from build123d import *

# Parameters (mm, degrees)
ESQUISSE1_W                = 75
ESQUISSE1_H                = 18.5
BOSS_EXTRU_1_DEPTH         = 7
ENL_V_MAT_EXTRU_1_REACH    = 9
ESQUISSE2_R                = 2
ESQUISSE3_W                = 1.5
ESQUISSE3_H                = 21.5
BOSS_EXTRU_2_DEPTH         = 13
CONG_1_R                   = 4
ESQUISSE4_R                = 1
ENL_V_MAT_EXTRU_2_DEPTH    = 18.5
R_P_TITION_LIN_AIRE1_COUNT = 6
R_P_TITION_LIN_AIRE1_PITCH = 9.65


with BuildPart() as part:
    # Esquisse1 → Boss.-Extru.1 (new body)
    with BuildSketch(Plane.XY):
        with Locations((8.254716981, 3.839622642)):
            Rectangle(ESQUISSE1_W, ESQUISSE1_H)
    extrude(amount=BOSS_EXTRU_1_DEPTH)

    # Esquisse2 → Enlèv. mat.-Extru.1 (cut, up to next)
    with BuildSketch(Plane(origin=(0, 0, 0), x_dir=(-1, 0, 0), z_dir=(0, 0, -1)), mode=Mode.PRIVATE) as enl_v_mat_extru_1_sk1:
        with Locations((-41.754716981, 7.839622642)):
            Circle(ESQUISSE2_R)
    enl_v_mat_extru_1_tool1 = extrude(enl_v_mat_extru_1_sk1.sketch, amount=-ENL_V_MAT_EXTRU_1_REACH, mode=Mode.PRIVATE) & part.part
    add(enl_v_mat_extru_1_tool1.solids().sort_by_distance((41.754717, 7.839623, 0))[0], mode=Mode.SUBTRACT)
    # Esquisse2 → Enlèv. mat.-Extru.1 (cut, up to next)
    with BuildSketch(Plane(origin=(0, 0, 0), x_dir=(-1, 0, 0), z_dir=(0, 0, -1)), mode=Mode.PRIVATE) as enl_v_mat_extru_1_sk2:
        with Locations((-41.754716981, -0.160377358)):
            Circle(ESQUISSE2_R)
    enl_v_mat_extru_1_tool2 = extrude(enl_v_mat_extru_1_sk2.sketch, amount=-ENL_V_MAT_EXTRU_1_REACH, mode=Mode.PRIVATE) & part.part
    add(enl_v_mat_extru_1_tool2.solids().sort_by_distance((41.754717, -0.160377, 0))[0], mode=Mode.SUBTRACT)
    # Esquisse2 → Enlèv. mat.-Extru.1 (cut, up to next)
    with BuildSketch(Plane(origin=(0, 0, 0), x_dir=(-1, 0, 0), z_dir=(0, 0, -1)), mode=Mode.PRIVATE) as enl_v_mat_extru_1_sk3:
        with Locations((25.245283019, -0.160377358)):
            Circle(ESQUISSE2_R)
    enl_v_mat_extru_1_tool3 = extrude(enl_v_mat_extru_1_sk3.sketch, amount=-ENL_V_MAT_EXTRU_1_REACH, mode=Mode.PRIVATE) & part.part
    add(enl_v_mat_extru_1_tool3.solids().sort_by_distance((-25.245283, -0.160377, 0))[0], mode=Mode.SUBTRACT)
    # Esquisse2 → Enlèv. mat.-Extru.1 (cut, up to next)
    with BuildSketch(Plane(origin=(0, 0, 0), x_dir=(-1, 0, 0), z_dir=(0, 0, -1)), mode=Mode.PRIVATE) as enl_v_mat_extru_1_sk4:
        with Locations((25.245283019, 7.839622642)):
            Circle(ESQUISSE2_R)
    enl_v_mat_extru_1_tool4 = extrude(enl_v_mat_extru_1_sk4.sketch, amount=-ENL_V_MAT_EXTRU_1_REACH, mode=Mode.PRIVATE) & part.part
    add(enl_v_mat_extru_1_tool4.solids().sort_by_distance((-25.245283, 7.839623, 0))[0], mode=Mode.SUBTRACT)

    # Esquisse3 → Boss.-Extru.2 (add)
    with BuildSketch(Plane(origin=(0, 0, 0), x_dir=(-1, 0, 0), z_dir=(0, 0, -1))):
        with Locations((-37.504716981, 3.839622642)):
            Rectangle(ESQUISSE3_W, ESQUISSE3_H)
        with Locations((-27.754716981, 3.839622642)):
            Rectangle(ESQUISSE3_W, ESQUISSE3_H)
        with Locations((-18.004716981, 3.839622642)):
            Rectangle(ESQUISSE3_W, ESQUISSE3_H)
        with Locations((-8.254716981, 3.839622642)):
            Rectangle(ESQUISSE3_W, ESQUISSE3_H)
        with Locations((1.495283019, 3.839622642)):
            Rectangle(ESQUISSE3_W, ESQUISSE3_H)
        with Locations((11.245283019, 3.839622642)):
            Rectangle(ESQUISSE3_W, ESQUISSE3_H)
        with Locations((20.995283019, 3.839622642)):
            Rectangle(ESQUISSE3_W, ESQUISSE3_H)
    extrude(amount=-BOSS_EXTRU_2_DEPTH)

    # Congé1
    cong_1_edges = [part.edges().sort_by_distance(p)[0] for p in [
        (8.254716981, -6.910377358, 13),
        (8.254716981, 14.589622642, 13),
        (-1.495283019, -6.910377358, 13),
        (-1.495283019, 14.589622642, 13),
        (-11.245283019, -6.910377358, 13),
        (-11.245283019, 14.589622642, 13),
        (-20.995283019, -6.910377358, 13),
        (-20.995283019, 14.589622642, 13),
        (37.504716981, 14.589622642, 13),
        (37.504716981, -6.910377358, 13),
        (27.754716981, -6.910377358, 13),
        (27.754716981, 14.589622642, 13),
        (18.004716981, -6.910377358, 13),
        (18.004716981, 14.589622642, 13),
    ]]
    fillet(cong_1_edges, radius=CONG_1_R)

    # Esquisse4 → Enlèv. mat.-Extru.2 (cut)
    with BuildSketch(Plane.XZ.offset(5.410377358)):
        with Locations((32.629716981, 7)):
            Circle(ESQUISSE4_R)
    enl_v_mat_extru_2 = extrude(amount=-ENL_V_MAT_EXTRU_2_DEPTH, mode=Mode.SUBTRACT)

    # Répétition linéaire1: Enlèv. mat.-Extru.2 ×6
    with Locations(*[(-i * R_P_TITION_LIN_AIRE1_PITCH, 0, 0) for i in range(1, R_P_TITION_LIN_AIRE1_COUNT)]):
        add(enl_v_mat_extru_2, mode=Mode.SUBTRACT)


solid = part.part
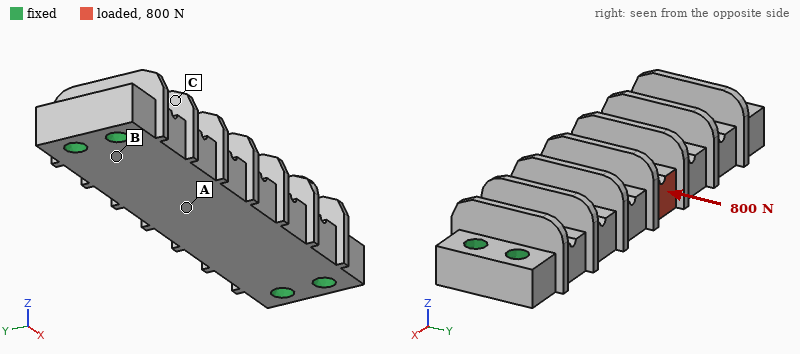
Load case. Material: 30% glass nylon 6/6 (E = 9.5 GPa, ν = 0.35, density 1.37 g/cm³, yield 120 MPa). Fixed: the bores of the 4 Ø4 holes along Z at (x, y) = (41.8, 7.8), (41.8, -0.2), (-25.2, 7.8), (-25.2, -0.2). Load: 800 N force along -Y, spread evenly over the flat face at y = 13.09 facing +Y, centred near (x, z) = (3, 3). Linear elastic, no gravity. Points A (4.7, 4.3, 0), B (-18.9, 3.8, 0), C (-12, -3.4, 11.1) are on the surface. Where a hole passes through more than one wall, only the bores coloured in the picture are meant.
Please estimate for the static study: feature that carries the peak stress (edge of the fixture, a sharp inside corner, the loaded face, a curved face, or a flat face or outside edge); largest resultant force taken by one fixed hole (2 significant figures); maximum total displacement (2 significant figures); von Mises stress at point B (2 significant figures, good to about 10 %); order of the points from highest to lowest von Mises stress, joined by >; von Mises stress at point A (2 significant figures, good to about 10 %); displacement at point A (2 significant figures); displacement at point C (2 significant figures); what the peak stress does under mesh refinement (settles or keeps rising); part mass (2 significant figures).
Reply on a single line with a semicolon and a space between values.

a sharp inside corner; 630 N; 76 µm; 12 MPa; B > A > C; 6.0 MPa; 68 µm; 34 µm; keeps rising; 15 g
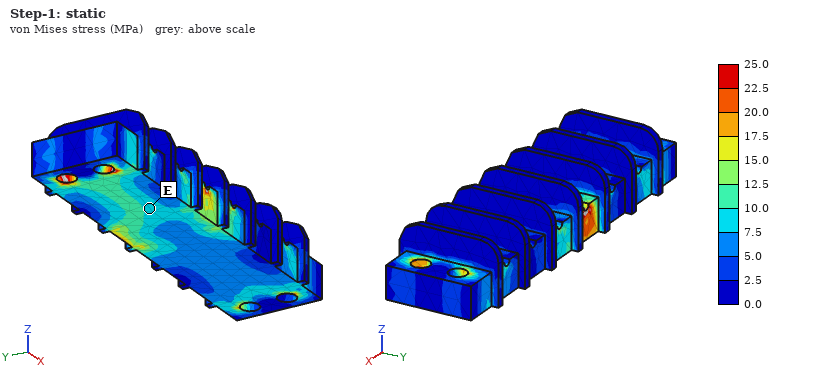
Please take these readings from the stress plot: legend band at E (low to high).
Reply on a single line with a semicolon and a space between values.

7.5 to 10.0 MPa
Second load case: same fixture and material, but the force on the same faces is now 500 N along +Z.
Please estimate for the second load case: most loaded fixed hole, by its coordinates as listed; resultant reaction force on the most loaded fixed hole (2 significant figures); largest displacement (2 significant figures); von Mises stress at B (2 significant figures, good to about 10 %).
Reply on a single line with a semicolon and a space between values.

(-25.2, 7.8); 320 N; 0.29 mm; 24 MPa
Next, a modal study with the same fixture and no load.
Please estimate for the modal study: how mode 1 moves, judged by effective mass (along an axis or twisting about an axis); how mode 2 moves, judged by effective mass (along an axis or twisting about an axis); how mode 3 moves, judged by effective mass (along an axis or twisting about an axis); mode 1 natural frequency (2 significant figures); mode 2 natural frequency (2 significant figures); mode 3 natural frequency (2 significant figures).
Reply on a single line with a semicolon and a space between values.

along Z; along Y; along Y; 3800 Hz; 6500 Hz; 7500 Hz
